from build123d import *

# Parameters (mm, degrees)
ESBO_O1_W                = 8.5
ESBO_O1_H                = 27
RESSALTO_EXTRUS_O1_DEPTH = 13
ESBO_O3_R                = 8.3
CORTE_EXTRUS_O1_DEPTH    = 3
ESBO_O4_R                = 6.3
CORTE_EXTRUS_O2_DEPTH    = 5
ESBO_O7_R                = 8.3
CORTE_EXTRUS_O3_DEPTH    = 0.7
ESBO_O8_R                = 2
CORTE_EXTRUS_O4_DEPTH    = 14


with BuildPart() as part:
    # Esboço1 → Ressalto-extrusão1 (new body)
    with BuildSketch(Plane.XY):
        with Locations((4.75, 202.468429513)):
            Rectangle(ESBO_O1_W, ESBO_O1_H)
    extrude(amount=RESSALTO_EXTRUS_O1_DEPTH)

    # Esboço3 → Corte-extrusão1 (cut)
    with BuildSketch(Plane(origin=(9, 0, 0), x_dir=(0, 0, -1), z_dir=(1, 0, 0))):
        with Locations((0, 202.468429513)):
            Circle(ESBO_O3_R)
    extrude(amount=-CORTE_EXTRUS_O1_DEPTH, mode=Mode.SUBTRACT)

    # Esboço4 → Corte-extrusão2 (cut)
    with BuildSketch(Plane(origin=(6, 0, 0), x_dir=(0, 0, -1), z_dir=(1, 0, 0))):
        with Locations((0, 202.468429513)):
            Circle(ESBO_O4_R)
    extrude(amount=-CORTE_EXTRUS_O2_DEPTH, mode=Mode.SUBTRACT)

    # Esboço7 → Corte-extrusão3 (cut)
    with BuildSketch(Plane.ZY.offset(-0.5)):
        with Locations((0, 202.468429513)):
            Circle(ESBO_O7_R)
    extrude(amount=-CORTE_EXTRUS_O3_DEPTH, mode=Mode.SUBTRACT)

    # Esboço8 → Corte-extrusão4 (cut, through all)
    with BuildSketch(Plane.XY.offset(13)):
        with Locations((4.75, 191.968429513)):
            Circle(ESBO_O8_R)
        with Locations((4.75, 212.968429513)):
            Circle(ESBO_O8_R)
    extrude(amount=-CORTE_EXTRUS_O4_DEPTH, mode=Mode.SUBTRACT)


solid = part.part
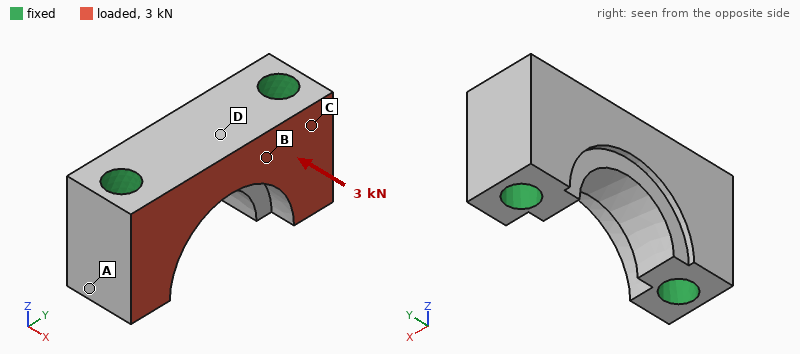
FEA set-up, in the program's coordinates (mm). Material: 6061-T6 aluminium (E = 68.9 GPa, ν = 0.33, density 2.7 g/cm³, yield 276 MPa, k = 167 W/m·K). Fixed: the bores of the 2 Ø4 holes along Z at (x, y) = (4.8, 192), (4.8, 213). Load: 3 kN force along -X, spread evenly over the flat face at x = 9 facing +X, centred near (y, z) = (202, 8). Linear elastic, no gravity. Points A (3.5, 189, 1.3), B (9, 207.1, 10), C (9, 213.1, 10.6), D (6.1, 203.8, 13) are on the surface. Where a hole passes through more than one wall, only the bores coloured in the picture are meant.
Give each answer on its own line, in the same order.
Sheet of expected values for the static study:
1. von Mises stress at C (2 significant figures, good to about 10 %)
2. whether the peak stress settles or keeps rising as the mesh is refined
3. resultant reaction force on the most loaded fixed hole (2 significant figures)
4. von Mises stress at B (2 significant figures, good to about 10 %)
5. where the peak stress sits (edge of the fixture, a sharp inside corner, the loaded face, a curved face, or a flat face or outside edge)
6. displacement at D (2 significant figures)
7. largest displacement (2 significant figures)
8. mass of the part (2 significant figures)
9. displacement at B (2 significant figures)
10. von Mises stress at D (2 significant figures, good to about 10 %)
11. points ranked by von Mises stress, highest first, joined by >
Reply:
22 MPa
keeps rising
1.5 kN
14 MPa
edge of the fixture
4.4 µm
5.0 µm
5.3 g
3.2 µm
9.2 MPa
C > B > D > A
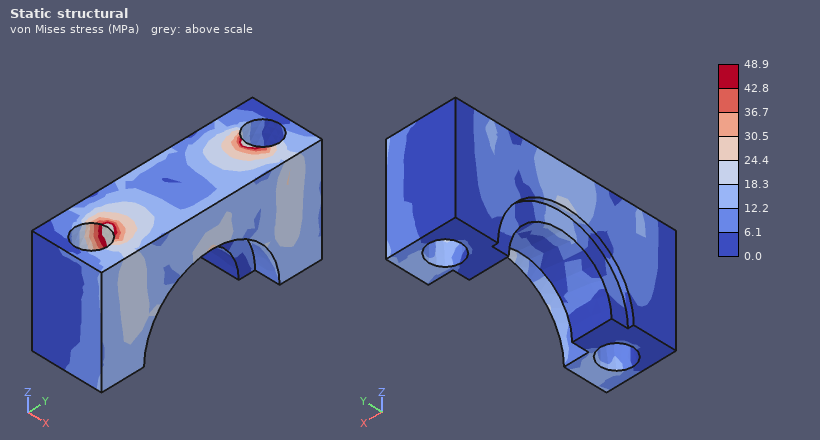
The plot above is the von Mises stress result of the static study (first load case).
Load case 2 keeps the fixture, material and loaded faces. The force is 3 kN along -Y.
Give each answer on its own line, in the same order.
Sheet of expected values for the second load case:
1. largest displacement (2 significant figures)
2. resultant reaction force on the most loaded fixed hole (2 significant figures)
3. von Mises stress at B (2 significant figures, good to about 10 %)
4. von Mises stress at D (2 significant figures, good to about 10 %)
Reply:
2.9 µm
1.5 kN
22 MPa
13 MPa
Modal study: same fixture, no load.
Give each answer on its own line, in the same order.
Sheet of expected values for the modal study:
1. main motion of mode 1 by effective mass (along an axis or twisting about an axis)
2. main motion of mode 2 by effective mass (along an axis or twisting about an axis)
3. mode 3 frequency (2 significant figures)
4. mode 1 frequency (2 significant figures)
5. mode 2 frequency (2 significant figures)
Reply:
along X
along Z
98 kHz
64 kHz
80 kHz
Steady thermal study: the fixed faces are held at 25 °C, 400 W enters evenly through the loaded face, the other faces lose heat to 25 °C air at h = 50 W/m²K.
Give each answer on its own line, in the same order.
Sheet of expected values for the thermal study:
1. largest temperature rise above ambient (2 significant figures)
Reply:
69 K
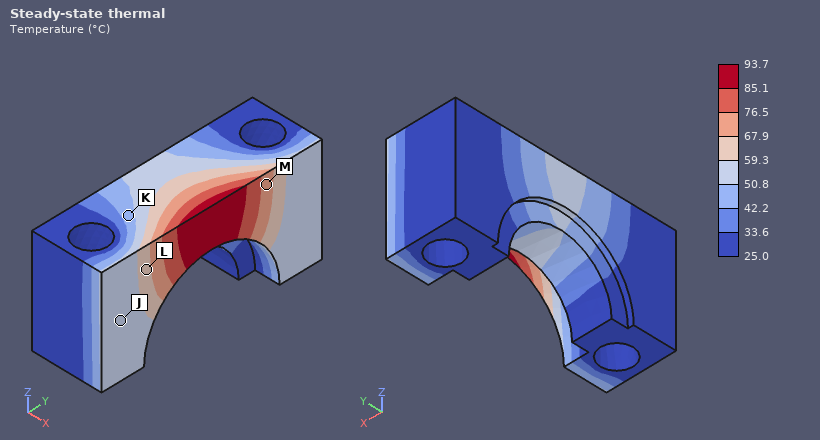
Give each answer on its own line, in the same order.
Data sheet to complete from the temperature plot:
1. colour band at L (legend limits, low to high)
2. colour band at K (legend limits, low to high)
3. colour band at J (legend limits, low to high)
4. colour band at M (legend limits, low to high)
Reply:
59.3 to 67.9 °C
42.2 to 50.8 °C
50.8 to 59.3 °C
67.9 to 76.5 °C
